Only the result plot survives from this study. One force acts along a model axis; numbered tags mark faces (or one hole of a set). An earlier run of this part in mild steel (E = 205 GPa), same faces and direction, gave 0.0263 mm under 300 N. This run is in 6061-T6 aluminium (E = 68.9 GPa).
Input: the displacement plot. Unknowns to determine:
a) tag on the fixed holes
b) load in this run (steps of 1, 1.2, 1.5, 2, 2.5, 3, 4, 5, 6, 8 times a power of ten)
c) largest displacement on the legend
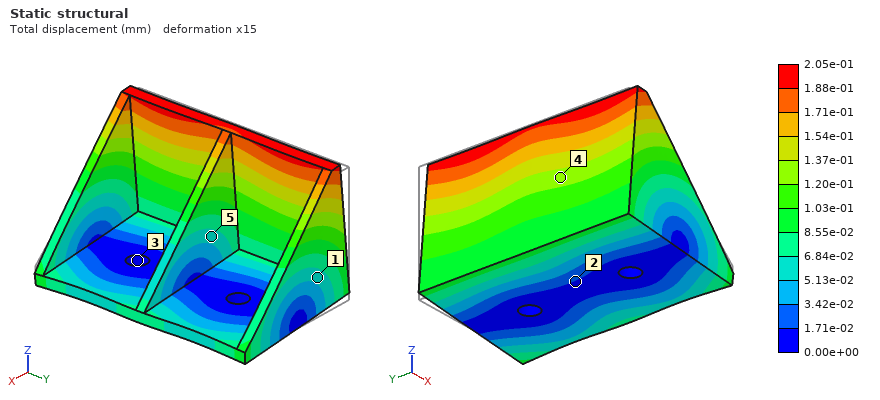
3
800 N
2.05e-01 mm
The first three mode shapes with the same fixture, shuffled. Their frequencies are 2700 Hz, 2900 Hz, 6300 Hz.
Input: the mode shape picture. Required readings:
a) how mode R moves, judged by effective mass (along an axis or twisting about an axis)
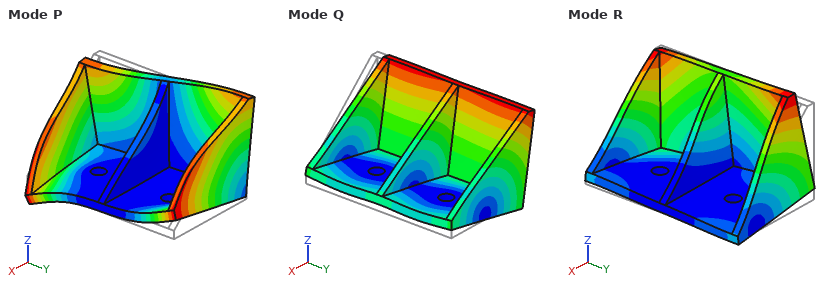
along Y
